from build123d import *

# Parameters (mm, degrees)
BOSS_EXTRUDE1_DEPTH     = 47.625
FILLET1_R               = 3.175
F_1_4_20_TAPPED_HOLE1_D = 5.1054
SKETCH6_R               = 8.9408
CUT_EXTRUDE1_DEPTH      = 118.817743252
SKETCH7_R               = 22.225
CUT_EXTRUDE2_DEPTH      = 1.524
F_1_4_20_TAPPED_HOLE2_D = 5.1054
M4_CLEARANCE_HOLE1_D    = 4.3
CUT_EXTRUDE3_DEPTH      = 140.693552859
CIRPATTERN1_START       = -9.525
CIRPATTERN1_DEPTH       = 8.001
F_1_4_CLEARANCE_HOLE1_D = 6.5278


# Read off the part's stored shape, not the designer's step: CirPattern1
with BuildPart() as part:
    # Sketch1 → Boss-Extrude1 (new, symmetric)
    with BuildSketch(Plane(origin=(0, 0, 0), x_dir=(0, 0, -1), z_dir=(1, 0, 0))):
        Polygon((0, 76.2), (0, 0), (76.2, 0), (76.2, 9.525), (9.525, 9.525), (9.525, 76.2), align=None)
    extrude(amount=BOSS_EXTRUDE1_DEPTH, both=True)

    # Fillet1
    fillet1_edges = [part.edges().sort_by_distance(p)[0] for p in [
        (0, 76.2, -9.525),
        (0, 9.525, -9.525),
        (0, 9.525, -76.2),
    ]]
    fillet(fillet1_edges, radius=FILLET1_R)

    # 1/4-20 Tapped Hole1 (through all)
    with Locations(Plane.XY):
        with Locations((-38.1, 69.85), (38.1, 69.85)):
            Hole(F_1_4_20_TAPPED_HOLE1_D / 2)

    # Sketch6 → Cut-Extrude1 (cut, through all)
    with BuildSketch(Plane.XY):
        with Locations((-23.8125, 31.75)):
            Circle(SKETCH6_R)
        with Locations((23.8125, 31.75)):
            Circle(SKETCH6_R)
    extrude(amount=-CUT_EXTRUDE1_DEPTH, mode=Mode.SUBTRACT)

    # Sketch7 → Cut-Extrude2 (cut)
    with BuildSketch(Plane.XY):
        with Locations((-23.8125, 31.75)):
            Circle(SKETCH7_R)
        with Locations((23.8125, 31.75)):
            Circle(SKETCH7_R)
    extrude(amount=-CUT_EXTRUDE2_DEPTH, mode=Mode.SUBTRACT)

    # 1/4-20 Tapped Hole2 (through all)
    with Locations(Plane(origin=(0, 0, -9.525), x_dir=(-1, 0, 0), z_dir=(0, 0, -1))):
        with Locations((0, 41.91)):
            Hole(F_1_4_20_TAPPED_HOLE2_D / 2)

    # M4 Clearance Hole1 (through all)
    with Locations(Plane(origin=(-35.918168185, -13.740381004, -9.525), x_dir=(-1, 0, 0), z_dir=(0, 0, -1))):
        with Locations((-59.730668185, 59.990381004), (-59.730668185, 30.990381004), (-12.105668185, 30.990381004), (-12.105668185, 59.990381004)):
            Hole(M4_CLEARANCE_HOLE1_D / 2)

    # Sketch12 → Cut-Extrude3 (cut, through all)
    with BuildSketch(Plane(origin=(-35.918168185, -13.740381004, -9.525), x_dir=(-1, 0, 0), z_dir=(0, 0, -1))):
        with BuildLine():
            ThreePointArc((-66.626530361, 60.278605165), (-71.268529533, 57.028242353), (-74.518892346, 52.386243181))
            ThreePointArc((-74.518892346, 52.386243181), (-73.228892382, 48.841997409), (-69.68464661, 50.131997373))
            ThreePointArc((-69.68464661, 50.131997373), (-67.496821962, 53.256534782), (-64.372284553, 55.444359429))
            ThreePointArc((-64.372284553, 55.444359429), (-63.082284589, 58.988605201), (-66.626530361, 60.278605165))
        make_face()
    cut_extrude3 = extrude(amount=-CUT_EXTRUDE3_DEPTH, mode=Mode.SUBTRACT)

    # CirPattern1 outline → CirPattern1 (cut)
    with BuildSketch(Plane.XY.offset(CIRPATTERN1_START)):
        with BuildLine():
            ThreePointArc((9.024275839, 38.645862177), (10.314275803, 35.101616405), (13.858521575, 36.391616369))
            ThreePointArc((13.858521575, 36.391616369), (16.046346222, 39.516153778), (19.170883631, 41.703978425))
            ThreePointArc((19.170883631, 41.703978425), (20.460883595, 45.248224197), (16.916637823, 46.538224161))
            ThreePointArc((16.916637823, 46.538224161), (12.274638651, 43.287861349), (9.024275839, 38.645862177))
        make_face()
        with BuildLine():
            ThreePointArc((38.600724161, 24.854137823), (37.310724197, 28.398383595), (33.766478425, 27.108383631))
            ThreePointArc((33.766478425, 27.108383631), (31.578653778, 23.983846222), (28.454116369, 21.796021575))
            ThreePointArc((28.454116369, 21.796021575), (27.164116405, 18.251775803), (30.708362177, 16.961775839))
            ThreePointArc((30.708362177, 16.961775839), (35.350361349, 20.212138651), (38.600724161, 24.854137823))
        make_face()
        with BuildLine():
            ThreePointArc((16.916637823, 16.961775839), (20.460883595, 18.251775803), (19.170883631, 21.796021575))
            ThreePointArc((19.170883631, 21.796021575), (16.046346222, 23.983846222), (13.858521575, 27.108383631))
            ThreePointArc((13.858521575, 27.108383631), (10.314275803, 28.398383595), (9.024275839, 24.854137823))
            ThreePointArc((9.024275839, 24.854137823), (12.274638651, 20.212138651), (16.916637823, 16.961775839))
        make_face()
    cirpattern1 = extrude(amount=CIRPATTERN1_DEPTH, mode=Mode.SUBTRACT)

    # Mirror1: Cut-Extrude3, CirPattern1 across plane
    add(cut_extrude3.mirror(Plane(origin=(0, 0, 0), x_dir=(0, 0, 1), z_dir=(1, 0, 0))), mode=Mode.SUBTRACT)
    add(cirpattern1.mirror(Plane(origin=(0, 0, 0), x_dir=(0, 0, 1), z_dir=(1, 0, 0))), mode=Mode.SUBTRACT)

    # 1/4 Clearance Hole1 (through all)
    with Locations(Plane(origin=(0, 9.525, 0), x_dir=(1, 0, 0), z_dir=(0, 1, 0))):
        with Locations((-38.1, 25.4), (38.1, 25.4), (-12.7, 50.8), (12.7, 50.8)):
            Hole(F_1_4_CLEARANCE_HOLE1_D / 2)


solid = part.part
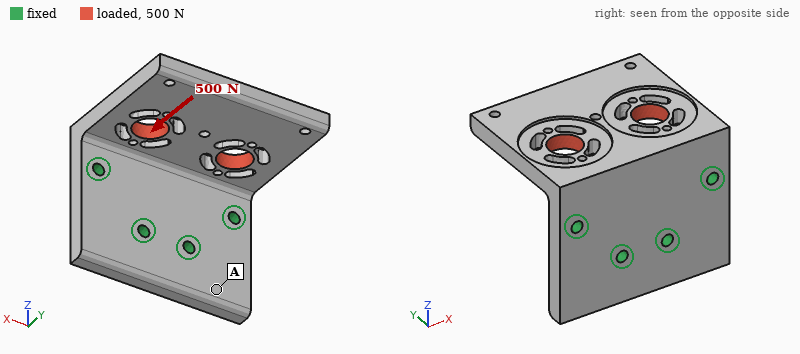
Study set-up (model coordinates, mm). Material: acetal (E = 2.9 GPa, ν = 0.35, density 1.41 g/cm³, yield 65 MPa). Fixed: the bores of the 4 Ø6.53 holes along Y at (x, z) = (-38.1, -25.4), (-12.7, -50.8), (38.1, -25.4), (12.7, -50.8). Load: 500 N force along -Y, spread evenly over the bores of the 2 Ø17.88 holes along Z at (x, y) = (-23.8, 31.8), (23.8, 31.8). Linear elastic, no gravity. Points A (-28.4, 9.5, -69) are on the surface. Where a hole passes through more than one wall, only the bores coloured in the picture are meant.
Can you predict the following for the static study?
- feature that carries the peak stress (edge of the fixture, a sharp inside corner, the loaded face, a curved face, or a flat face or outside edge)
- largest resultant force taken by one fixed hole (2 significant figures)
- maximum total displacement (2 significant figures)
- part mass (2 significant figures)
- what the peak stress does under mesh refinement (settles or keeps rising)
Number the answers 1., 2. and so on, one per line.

1. edge of the fixture
2. 280 N
3. 0.45 mm
4. 160 g
5. keeps rising
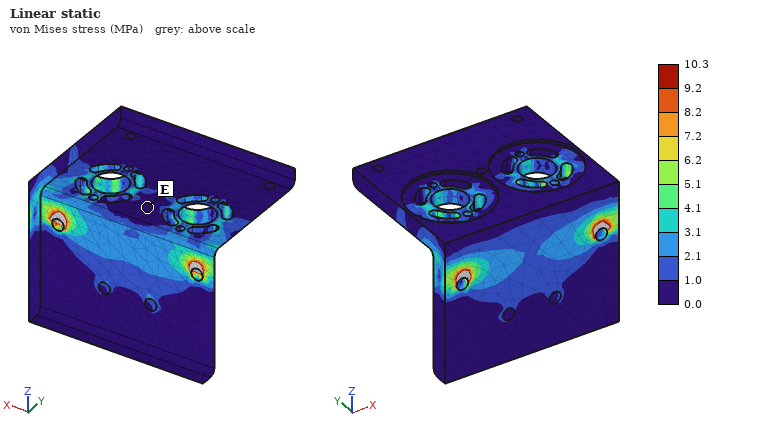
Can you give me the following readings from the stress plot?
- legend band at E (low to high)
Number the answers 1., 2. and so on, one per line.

1. 0.0 to 1.0 MPa
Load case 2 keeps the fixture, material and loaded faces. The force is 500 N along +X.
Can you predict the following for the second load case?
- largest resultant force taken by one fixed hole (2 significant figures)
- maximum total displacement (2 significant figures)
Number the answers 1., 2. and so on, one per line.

1. 310 N
2. 0.22 mm
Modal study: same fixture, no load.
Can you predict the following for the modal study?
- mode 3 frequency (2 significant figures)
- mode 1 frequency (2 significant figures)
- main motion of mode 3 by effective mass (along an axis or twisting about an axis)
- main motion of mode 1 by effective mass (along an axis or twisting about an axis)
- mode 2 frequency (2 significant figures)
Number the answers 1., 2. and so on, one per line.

1. 950 Hz
2. 260 Hz
3. along X
4. along Z
5. 600 Hz
